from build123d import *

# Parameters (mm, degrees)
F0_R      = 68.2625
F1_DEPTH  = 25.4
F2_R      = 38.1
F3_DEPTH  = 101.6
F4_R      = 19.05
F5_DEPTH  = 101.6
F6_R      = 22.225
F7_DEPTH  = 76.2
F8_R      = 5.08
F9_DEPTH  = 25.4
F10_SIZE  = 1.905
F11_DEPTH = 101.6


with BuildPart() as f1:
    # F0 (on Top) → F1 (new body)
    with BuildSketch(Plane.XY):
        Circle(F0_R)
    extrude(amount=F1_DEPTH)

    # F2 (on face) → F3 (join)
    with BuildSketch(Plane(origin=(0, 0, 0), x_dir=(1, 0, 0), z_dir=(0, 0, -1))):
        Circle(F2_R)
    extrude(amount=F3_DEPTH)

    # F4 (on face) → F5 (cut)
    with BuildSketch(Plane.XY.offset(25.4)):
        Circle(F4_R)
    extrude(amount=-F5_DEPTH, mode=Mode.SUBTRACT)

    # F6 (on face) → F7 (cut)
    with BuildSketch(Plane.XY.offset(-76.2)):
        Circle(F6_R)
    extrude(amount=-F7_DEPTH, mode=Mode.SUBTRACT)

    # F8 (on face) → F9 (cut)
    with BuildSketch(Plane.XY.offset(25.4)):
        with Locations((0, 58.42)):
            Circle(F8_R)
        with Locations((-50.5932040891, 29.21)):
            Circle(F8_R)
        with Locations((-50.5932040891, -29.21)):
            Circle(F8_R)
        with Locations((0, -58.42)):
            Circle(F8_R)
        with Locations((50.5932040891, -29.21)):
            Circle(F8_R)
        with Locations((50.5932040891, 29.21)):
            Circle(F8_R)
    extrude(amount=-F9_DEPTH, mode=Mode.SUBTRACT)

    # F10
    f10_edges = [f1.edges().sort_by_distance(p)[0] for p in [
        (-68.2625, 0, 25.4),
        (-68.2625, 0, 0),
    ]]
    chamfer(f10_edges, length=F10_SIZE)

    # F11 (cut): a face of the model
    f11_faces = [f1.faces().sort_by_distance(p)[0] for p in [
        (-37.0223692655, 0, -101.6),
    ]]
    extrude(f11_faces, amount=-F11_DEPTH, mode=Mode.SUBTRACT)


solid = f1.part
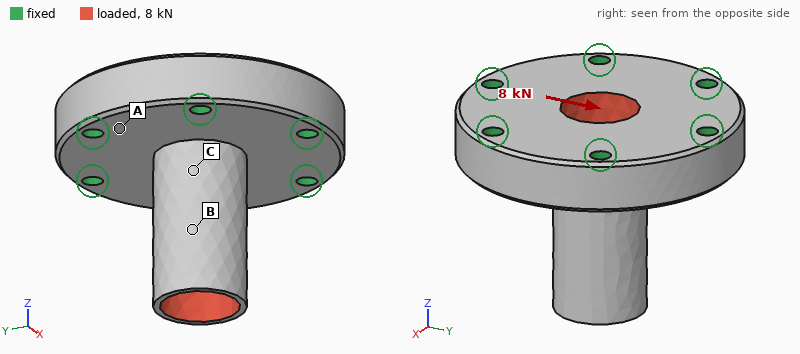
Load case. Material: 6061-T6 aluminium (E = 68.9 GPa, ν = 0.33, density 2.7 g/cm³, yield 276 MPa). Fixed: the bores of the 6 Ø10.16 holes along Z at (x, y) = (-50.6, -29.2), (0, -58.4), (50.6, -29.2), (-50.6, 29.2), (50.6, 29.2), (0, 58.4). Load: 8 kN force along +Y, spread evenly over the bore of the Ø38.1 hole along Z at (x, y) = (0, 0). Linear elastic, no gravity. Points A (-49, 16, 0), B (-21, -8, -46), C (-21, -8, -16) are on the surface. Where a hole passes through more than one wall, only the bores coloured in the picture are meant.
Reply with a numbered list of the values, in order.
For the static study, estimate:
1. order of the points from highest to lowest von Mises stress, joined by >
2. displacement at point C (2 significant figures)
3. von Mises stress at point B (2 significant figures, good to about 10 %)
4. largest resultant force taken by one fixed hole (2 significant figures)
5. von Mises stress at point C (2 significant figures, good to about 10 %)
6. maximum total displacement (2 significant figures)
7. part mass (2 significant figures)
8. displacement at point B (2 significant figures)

1. C > B > A
2. 0.030 mm
3. 18 MPa
4. 3.0 kN
5. 36 MPa
6. 0.14 mm
7. 970 g
8. 0.085 mm
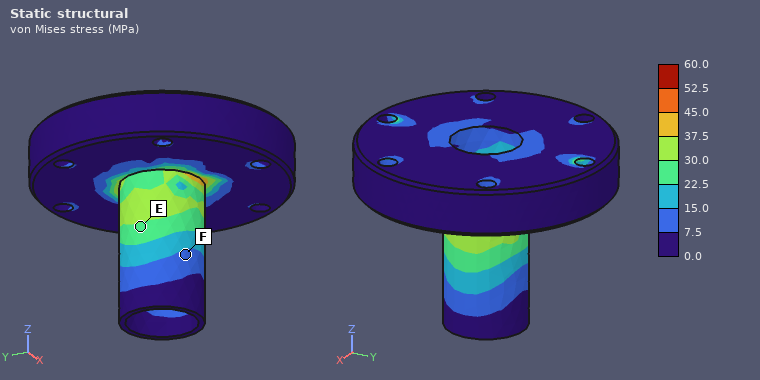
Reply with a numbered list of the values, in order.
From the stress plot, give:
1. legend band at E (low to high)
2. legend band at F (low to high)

1. 22.5 to 30.0 MPa
2. 7.5 to 15.0 MPa
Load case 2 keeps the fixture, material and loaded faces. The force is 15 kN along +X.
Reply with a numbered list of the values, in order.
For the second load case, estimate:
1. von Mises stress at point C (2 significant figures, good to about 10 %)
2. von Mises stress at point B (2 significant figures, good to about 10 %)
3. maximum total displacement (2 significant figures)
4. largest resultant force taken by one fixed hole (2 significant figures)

1. 61 MPa
2. 22 MPa
3. 0.26 mm
4. 5.0 kN
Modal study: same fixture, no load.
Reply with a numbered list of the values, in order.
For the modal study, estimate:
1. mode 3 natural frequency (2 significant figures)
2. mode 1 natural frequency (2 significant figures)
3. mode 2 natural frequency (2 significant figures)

1. 5600 Hz
2. 4200 Hz
3. 4300 Hz
